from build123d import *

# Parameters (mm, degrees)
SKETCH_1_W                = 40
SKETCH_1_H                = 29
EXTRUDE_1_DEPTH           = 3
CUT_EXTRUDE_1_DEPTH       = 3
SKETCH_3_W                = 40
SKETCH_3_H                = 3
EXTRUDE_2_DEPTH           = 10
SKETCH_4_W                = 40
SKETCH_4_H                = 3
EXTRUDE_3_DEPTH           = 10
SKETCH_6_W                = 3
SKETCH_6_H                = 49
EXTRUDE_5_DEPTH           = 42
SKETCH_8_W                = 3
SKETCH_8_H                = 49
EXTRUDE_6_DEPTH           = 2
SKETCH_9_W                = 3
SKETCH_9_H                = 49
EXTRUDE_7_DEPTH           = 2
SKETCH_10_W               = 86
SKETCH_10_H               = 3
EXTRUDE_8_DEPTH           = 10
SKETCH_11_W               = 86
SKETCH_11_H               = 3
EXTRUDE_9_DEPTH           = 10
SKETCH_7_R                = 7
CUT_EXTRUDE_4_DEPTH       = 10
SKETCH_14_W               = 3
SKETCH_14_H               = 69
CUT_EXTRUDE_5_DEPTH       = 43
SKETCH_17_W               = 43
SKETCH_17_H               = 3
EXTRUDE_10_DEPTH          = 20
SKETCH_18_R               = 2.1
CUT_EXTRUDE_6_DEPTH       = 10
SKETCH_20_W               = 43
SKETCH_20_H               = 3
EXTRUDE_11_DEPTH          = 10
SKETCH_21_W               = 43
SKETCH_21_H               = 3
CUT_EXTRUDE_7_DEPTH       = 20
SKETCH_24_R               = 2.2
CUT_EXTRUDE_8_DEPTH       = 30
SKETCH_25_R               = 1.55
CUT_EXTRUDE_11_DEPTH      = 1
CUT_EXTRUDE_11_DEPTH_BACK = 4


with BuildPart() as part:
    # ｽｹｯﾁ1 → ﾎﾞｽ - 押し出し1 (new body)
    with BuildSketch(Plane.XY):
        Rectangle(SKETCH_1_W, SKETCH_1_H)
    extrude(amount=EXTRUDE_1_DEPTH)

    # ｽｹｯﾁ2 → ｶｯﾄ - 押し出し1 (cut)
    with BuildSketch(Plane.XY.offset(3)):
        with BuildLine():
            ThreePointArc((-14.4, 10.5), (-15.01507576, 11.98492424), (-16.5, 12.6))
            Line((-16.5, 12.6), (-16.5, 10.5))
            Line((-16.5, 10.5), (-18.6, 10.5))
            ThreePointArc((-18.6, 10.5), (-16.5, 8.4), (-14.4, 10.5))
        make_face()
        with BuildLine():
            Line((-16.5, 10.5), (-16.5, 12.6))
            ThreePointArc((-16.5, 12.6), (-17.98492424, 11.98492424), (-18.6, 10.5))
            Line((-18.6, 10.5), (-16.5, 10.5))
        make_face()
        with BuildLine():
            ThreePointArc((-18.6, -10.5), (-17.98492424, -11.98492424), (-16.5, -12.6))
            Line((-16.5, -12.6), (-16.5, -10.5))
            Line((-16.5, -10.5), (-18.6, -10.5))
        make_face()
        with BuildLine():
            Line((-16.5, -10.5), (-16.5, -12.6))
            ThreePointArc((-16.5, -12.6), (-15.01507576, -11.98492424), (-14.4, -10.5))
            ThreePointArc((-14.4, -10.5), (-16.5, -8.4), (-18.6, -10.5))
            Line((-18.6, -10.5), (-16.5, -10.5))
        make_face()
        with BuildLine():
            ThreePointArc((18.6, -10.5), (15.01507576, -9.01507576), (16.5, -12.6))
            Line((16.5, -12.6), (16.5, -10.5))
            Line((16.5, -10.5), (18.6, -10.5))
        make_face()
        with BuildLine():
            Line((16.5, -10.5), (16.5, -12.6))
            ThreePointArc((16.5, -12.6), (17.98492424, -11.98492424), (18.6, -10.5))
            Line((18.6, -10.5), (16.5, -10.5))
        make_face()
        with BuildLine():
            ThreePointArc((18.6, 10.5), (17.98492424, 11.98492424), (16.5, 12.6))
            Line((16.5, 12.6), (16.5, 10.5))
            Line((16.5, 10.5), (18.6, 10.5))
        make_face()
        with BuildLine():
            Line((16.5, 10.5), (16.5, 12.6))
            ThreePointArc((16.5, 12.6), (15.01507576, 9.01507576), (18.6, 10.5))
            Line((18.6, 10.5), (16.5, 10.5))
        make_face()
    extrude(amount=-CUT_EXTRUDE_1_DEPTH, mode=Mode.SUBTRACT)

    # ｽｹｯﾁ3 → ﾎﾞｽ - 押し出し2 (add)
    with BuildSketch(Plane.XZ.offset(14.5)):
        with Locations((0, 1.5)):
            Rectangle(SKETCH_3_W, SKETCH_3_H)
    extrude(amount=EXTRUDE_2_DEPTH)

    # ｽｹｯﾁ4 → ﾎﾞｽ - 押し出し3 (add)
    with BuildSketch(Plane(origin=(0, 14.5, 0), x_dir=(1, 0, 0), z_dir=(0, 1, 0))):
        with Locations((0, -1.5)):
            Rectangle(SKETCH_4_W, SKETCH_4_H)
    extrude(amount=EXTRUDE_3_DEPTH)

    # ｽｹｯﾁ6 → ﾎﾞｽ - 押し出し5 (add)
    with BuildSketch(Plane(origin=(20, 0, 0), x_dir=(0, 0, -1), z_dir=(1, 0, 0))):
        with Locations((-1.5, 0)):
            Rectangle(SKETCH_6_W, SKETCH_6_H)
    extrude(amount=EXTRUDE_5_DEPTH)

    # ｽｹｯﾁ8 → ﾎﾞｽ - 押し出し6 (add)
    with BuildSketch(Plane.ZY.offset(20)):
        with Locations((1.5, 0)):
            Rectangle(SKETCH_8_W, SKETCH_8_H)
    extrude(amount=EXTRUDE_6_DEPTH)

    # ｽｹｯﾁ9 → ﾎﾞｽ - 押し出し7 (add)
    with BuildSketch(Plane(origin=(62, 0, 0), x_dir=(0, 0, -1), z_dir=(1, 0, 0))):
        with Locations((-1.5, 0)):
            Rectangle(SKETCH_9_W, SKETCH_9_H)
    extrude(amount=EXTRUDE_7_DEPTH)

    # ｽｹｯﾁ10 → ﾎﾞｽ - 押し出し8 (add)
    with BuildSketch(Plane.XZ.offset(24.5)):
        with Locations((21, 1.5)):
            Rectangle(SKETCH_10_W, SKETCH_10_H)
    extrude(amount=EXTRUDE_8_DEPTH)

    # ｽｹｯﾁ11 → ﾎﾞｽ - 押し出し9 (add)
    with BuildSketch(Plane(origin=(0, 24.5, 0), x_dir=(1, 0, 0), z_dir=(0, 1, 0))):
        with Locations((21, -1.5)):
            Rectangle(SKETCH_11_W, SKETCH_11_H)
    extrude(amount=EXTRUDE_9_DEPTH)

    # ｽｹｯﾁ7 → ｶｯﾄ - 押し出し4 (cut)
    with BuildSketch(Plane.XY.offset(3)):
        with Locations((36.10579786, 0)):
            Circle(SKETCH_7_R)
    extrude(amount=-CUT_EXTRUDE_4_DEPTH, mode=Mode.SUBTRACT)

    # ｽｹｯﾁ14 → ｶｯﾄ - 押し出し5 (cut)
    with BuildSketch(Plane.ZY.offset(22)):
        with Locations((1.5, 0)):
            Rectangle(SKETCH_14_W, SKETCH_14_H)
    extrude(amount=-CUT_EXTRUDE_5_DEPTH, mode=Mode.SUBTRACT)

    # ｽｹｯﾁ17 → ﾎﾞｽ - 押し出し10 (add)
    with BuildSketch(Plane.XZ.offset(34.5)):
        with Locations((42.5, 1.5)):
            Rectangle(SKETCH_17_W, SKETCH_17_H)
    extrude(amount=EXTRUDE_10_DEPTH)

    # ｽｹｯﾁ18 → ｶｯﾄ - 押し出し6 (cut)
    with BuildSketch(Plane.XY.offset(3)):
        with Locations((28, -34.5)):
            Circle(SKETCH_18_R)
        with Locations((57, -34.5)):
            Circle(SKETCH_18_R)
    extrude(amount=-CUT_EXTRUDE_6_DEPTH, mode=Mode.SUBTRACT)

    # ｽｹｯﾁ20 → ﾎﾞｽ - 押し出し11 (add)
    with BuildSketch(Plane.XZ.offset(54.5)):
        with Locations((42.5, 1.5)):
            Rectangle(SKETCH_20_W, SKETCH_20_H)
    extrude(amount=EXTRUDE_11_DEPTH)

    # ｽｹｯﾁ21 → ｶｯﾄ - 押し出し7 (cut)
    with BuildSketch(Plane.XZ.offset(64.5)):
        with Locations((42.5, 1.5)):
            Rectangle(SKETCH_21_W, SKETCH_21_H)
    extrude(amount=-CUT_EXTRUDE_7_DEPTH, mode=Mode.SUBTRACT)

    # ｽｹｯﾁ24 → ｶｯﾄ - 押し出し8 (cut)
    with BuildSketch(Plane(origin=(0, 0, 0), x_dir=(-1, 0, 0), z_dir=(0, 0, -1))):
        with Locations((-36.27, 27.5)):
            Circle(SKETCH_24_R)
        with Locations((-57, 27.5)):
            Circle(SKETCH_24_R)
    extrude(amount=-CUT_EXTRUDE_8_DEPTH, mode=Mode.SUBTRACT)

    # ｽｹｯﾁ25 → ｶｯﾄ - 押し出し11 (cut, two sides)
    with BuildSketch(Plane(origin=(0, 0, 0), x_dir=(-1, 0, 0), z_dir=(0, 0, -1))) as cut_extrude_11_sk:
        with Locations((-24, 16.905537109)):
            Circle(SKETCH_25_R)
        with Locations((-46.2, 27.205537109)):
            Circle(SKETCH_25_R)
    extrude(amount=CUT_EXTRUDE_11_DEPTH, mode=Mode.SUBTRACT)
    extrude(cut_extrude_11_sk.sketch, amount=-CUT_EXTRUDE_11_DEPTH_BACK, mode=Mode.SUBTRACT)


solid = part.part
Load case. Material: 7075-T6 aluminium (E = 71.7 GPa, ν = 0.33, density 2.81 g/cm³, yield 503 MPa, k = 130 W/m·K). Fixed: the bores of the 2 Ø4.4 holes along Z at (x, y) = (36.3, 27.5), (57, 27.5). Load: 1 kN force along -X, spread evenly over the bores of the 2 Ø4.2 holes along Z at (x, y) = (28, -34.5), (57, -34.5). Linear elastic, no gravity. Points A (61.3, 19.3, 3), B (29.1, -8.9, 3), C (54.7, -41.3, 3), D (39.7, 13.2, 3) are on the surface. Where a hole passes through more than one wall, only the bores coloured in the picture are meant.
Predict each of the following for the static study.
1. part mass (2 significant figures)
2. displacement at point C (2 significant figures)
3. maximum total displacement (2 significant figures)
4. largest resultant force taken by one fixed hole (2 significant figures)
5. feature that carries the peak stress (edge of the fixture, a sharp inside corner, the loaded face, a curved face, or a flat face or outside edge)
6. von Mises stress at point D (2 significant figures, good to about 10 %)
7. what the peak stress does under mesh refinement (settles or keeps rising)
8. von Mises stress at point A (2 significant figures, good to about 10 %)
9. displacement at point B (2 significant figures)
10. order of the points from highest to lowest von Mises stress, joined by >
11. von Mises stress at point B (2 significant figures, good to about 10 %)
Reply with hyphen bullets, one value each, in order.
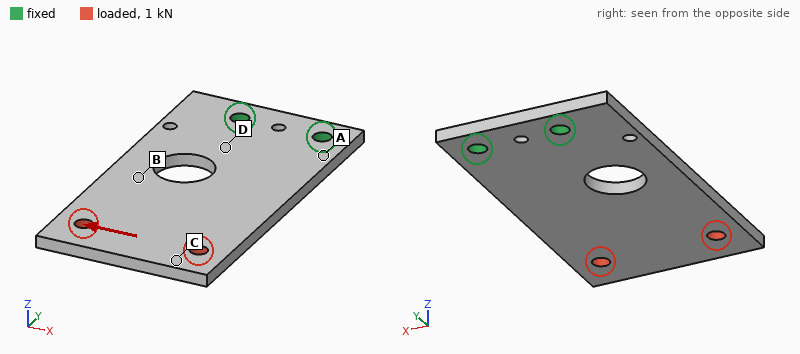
- 27 g
- 0.14 mm
- 0.15 mm
- 2.7 kN
- edge of the fixture
- 47 MPa
- keeps rising
- 63 MPa
- 0.073 mm
- A > D > B > C
- 31 MPa
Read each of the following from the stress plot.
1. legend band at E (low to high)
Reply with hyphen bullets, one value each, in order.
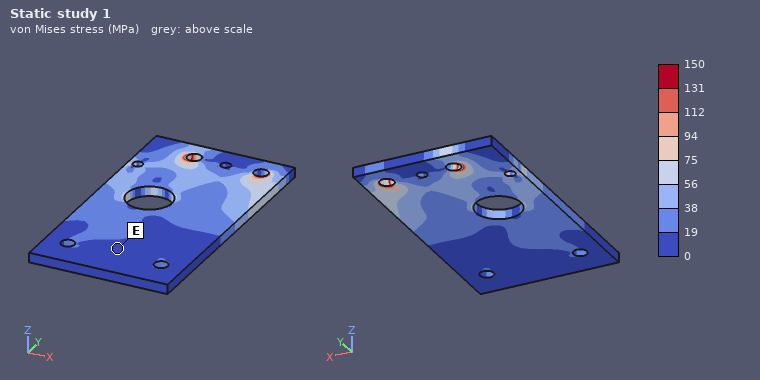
- 0 to 19 MPa
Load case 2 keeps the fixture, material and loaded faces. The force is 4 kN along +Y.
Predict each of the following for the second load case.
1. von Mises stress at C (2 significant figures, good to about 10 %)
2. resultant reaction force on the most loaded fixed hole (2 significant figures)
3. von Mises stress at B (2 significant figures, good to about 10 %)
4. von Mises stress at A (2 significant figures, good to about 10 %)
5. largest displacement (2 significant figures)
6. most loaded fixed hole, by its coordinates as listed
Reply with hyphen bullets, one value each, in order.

- 21 MPa
- 2.7 kN
- 42 MPa
- 28 MPa
- 64 µm
- (36.3, 27.5)
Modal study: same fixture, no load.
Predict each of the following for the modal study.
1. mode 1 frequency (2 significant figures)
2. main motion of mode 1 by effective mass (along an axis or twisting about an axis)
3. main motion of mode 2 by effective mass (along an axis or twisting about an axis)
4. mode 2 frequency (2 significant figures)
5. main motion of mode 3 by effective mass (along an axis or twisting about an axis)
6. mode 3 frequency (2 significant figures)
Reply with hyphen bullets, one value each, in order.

- 460 Hz
- along Z
- twisting about Y
- 1600 Hz
- along Z
- 2900 Hz
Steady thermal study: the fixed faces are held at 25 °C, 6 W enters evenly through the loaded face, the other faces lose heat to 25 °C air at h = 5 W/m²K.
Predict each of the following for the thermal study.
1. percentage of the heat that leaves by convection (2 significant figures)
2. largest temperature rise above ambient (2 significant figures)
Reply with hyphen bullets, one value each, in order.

- 7.8 %
- 26 K
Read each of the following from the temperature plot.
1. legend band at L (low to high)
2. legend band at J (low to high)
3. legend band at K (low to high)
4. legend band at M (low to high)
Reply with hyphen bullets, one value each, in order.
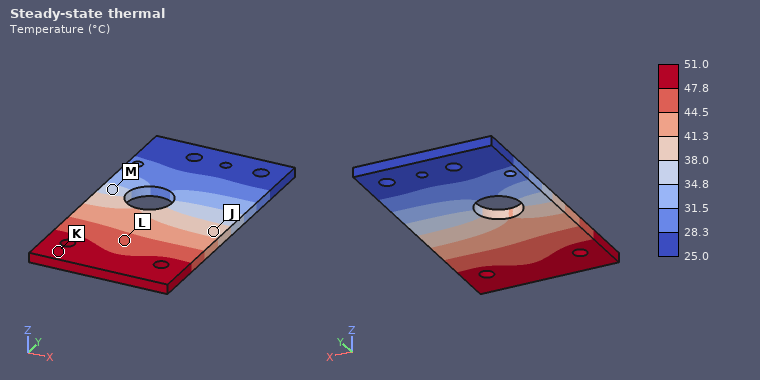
- 44.5 to 47.8 °C
- 38.0 to 41.3 °C
- 47.8 to 51.0 °C
- 34.8 to 38.0 °C
